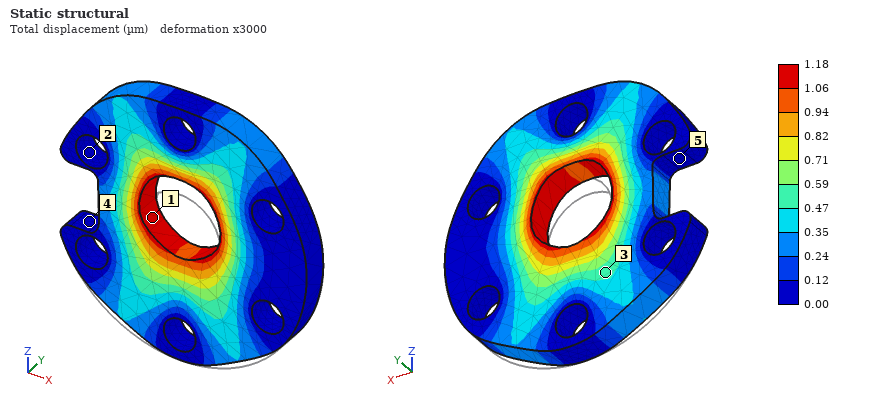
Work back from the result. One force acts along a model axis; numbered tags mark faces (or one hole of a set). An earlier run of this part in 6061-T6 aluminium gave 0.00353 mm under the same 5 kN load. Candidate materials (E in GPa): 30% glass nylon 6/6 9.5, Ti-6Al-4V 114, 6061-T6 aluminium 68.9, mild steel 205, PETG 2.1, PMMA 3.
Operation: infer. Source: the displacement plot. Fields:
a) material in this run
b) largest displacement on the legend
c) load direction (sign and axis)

mild steel
1.18 µm
+Z
